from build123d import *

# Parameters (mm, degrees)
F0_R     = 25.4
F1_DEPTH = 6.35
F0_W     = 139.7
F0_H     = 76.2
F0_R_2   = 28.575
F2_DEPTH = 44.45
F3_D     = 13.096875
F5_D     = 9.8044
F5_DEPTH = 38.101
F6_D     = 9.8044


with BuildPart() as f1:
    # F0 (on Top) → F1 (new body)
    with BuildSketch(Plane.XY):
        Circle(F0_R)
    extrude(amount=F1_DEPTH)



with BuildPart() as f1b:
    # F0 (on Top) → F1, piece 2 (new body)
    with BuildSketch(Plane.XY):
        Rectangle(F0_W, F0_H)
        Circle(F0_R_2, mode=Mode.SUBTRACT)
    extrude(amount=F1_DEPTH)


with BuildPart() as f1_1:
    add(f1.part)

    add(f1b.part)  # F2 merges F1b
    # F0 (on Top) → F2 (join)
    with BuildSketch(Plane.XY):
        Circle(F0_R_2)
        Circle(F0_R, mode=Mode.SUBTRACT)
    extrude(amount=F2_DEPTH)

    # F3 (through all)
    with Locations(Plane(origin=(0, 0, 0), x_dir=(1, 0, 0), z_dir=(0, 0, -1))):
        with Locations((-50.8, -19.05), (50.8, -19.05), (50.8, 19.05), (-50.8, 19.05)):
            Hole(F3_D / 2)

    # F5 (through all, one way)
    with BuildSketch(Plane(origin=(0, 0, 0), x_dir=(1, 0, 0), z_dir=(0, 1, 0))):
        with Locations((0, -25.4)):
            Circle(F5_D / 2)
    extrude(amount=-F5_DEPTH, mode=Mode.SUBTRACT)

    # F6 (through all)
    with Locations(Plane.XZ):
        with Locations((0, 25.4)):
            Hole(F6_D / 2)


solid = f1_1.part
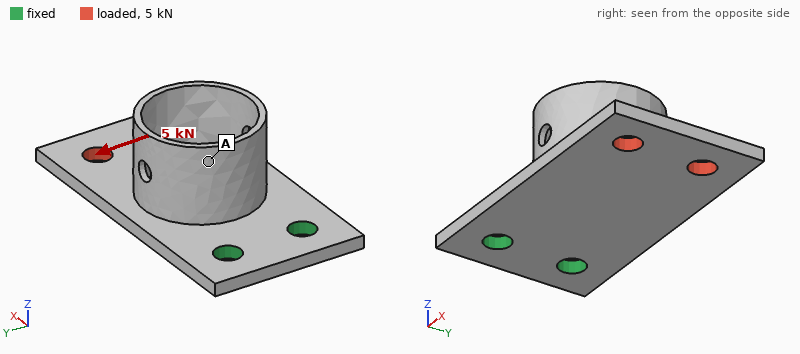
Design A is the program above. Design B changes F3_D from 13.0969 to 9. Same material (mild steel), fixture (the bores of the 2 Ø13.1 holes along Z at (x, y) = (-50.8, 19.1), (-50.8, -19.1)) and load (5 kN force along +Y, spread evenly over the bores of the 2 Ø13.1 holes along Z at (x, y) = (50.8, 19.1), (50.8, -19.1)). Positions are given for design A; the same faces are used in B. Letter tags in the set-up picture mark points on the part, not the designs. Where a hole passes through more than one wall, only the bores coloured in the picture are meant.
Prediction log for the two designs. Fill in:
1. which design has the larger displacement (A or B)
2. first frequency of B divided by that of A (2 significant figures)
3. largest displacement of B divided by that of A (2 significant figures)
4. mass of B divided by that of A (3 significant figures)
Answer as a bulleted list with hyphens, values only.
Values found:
- B
- 0.93
- 1.1
- 1.02
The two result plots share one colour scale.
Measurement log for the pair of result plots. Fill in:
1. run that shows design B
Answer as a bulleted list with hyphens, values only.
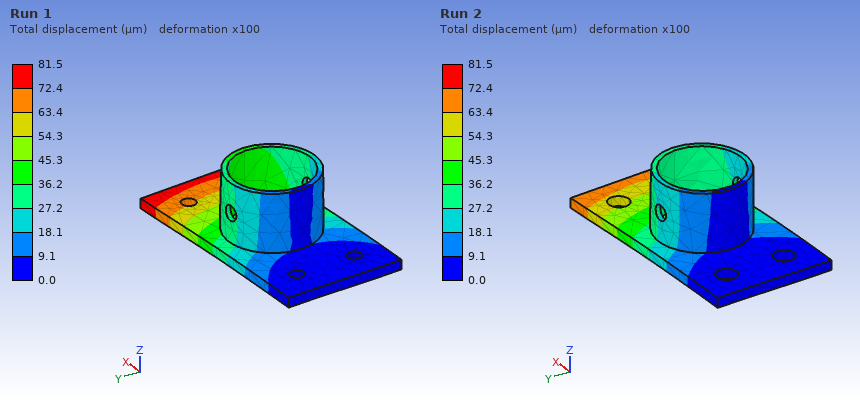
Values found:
- Run 1
